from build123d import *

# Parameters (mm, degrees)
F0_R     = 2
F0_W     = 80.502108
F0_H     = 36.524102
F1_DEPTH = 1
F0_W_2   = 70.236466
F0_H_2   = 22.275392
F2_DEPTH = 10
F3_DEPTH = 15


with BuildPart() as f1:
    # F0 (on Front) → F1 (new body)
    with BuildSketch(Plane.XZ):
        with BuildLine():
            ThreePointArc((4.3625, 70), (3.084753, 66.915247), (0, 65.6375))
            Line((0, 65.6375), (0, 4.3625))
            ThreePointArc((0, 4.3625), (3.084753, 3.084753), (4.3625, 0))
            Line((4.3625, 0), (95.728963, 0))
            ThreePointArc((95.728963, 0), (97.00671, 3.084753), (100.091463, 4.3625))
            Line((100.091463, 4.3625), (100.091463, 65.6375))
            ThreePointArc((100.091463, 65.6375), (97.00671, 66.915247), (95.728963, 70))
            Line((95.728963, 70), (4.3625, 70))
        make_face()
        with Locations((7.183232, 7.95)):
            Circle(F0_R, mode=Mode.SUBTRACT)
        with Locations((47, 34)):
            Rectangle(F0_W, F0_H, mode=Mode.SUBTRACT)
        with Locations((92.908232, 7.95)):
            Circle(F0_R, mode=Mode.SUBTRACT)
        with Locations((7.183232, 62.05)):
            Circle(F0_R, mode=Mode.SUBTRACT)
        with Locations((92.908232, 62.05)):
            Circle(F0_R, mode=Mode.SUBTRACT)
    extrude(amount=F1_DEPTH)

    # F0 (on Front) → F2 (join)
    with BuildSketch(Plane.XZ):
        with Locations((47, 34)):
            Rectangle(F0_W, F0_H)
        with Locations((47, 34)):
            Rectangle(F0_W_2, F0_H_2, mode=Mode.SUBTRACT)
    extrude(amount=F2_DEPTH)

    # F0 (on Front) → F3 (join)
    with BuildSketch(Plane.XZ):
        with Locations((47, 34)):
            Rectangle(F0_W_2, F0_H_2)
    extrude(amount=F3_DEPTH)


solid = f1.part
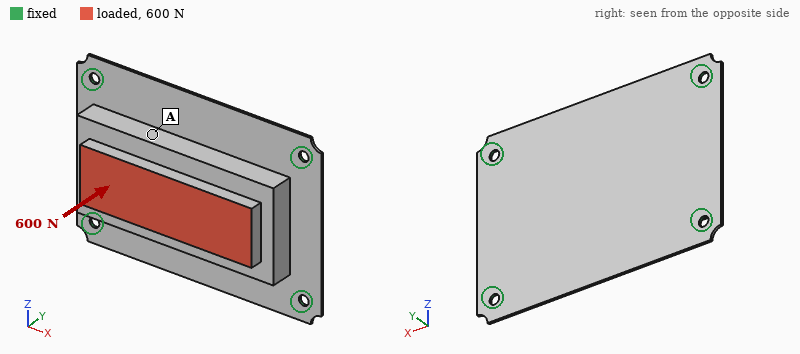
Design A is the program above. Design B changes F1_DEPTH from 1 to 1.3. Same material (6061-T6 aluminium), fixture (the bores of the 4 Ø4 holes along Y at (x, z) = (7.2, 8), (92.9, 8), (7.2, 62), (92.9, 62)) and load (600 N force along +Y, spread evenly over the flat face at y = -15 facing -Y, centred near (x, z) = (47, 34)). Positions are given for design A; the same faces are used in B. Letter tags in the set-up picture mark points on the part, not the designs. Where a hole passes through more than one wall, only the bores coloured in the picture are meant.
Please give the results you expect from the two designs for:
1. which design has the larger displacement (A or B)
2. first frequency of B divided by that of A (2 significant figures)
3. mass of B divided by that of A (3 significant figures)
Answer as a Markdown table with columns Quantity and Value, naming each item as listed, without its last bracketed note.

| Quantity | Value |
|---|---|
| which design has the larger displacement | A |
| first frequency of B divided by that of A | 1.3 |
| mass of B divided by that of A | 1.03 |
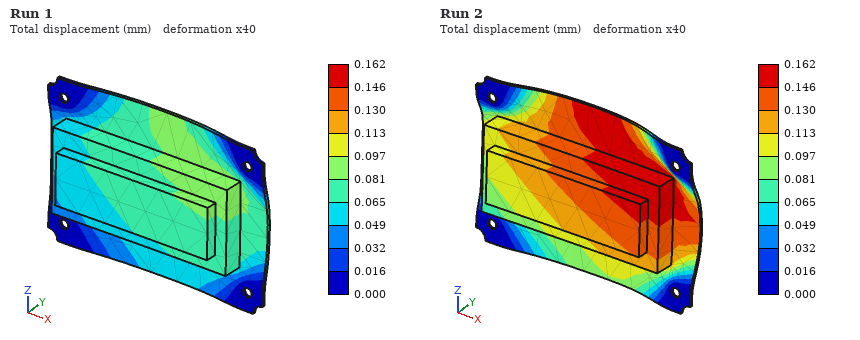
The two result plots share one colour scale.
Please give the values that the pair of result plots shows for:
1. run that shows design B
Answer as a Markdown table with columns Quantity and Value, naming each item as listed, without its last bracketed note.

| Quantity | Value |
|---|---|
| run that shows design B | Run 1 |
